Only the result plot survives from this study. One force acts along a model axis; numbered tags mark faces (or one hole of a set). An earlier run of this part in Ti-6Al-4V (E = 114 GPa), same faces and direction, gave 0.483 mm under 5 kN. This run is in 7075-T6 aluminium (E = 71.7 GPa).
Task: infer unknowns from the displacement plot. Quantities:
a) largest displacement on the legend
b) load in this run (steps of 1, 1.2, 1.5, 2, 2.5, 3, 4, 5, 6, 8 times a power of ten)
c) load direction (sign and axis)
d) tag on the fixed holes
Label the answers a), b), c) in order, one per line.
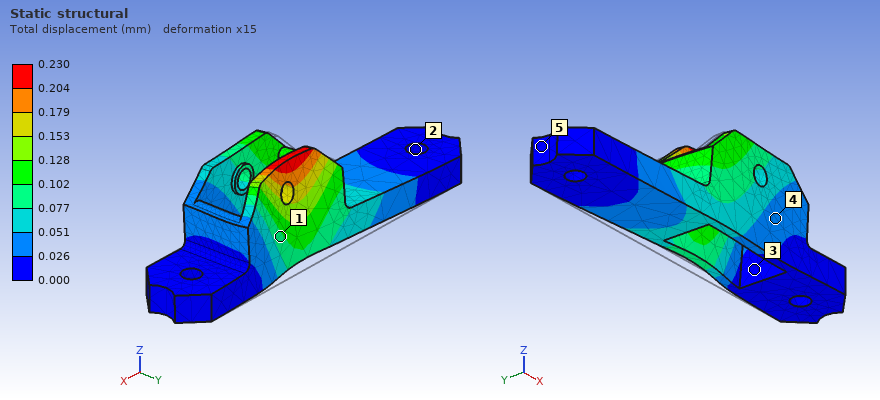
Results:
a) 0.230 mm
b) 1.5 kN
c) -Y
d) 2
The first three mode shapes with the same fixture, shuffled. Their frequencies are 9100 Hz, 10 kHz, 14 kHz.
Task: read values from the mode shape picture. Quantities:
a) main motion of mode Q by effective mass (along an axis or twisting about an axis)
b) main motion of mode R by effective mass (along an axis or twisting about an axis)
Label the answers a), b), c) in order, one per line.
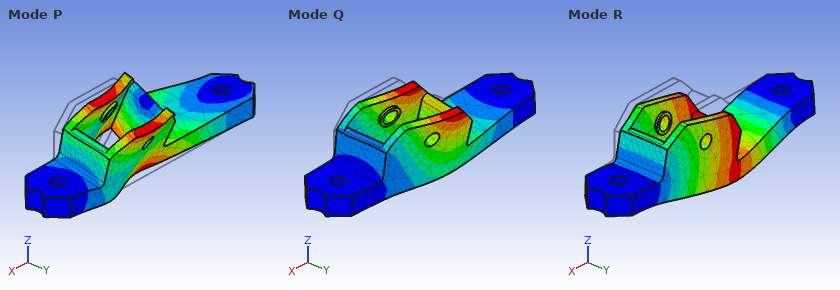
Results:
a) along Y
b) along Z
